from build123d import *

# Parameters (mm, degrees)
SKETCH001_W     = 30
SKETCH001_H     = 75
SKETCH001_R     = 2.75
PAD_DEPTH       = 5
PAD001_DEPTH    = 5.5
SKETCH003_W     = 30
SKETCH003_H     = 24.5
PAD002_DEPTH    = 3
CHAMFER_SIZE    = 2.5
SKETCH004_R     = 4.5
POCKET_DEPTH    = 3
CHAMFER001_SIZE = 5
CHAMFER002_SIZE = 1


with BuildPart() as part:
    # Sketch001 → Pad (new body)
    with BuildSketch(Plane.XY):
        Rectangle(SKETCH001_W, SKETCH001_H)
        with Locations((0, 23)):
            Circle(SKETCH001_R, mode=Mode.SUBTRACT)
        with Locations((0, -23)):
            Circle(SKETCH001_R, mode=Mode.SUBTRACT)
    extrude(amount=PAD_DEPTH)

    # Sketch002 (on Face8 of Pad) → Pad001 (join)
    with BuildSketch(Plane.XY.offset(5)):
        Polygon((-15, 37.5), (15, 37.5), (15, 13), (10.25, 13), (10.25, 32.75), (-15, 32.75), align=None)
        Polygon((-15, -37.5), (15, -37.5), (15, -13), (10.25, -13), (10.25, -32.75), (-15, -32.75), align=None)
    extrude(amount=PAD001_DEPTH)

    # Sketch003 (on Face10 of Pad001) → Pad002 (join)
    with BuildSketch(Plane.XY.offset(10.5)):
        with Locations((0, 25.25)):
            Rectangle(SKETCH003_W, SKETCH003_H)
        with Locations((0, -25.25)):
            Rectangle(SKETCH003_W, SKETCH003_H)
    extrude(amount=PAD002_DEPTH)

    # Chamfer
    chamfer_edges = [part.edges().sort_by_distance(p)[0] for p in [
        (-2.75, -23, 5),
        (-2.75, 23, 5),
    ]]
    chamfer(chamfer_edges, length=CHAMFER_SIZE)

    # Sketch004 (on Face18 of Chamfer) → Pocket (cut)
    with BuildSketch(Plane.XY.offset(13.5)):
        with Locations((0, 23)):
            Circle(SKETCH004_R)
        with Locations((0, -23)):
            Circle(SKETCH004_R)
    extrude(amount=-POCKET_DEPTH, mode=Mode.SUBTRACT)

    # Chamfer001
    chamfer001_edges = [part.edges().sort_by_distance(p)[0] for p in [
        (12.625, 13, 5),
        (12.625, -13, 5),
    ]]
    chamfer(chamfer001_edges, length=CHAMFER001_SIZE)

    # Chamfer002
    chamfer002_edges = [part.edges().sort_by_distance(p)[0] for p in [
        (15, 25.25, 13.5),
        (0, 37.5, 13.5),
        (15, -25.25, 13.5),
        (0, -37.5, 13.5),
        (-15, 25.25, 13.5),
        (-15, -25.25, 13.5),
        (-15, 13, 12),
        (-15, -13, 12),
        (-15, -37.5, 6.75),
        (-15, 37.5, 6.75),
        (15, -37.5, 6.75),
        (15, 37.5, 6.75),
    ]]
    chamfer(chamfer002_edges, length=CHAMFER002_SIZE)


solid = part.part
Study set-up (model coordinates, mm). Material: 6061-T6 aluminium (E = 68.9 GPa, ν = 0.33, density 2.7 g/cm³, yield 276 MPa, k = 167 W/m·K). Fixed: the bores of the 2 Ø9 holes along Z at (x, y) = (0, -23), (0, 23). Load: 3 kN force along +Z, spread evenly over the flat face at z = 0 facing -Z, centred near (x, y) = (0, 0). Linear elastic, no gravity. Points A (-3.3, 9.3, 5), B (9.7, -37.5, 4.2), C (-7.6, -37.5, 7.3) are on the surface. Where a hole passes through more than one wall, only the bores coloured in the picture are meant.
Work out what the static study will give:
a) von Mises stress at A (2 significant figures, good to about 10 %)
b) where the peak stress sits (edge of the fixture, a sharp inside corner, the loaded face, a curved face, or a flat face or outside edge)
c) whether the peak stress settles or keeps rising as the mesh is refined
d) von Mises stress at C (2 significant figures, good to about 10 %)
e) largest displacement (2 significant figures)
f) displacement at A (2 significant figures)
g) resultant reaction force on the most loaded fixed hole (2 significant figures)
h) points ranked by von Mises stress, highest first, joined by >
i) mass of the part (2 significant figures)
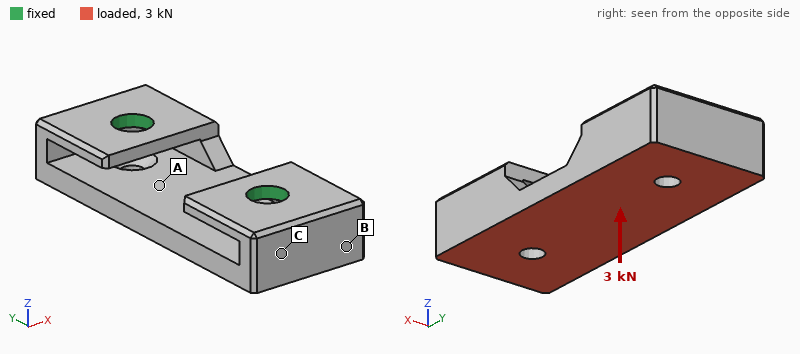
30 MPa
edge of the fixture
keeps rising
51 MPa
0.18 mm
0.099 mm
1.7 kN
C > A > B
47 g
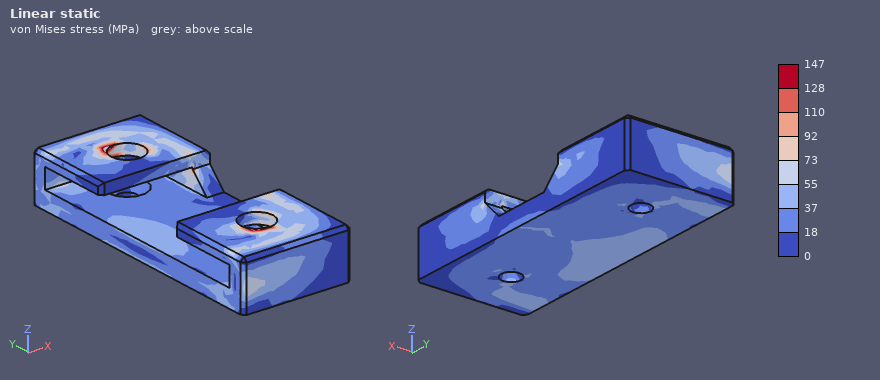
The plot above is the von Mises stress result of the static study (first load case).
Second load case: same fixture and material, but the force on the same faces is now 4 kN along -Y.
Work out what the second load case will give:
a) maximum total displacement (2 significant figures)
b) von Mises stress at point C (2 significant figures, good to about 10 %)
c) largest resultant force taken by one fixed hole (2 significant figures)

92 µm
23 MPa
2.1 kN
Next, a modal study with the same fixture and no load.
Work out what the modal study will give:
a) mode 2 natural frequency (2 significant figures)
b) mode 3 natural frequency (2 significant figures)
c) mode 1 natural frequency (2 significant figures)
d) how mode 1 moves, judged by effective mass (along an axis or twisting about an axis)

6600 Hz
6600 Hz
3900 Hz
along X
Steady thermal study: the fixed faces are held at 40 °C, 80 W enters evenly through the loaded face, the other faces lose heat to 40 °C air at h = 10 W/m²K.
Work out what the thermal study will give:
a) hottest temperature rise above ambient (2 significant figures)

43 K
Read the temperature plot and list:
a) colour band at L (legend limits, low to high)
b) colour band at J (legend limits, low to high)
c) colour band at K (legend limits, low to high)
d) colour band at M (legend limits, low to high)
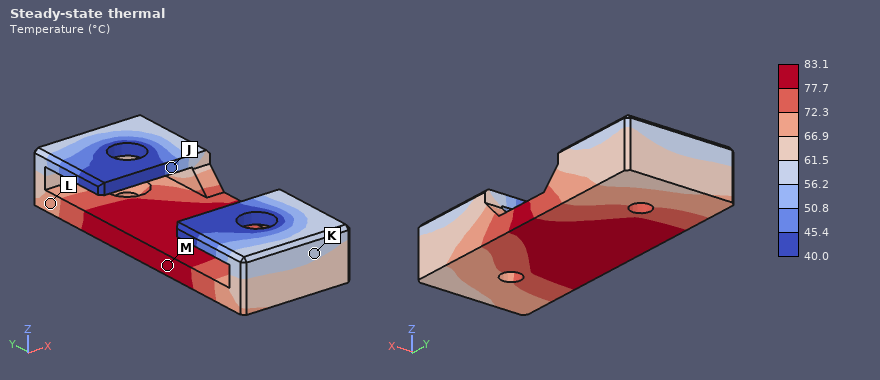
66.9 to 72.3 °C
45.4 to 50.8 °C
56.2 to 61.5 °C
77.7 to 83.1 °C
